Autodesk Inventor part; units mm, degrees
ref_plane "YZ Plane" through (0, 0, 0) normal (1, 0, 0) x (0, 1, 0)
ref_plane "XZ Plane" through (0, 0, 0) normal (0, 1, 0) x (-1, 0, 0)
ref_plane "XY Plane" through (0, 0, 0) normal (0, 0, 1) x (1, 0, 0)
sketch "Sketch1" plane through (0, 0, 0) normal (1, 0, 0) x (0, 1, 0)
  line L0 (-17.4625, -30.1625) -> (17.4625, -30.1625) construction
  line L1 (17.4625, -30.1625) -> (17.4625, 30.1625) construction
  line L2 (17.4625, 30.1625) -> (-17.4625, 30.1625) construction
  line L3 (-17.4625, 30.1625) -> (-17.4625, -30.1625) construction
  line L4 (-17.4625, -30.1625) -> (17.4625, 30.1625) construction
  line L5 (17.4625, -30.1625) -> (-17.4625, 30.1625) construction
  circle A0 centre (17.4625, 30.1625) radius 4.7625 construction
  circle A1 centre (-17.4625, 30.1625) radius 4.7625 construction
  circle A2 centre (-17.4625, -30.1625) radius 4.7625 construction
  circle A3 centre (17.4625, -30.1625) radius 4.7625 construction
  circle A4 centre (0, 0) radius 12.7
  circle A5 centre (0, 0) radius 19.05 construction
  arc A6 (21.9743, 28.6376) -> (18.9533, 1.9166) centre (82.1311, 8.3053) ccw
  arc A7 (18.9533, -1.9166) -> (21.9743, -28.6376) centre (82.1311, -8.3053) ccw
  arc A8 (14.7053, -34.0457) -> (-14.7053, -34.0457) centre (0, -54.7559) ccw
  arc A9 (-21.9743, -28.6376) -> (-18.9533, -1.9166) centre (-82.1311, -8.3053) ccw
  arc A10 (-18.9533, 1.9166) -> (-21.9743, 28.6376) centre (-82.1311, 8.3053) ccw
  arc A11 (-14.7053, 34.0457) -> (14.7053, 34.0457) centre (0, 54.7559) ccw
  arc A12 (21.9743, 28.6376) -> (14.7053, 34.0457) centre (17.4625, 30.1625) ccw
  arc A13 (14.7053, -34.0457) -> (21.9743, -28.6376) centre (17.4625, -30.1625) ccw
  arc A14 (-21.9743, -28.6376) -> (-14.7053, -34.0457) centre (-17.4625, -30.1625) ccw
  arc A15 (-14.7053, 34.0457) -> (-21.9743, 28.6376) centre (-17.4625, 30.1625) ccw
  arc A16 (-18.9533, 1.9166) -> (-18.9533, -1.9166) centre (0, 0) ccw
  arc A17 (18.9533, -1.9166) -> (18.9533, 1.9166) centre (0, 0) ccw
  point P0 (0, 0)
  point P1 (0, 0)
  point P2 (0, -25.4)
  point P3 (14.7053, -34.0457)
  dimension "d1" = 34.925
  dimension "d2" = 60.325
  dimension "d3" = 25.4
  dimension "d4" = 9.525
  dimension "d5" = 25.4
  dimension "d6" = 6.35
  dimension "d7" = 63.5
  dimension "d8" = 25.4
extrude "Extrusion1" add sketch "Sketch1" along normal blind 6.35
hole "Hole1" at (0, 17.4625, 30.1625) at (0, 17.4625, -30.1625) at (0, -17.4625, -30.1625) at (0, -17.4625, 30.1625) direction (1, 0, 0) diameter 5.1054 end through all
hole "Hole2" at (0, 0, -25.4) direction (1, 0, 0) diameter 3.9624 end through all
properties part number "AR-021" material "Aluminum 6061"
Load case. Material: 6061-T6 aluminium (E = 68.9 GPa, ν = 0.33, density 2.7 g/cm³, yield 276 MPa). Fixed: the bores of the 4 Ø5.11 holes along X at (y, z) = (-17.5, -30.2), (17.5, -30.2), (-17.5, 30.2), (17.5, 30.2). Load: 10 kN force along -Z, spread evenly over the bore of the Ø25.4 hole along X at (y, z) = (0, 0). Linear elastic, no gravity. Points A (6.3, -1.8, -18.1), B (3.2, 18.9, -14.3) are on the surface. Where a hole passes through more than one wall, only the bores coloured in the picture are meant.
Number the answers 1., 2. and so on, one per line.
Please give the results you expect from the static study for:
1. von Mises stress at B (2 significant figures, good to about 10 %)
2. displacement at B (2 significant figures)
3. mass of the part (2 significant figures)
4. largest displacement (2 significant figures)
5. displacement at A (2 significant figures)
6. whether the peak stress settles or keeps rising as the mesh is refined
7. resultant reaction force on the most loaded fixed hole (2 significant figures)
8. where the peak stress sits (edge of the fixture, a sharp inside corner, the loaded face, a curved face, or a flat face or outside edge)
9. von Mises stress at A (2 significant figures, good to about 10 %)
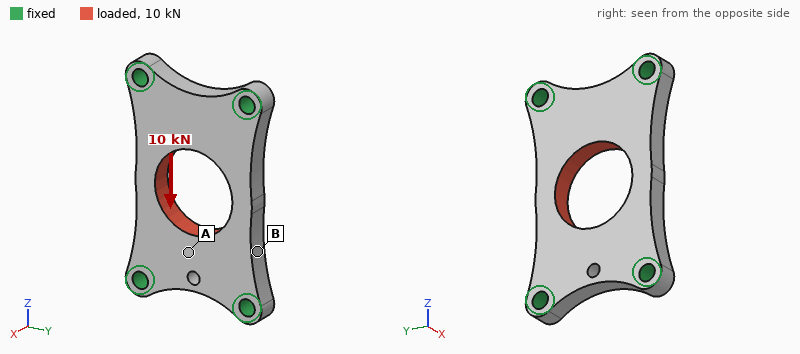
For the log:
1. 29 MPa
2. 6.0 µm
3. 33 g
4. 11 µm
5. 9.8 µm
6. keeps rising
7. 2.7 kN
8. edge of the fixture
9. 15 MPa
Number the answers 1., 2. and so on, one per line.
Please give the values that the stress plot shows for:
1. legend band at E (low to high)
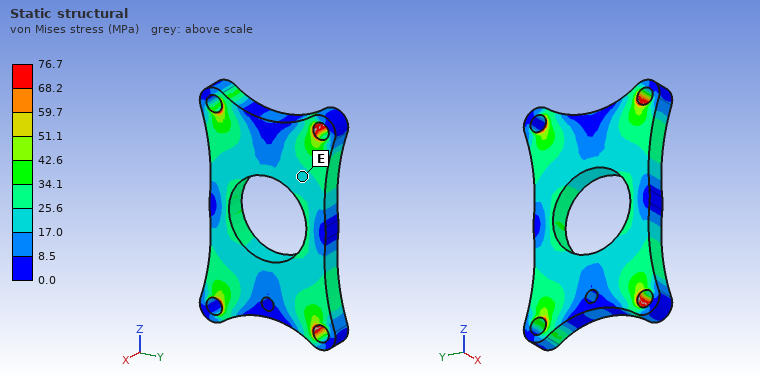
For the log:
1. 17.0 to 25.6 MPa
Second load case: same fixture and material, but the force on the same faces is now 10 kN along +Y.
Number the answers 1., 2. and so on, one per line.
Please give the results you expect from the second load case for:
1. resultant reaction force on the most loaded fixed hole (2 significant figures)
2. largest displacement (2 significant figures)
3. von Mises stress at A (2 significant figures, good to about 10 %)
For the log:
1. 3.2 kN
2. 38 µm
3. 68 MPa
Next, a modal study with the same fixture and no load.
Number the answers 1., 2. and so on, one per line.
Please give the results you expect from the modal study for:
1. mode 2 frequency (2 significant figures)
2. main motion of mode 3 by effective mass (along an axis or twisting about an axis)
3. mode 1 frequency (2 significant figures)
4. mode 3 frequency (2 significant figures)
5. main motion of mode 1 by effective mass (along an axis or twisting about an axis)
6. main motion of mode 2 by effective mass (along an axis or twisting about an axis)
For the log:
1. 12 kHz
2. twisting about Y
3. 8900 Hz
4. 16 kHz
5. along X
6. twisting about Z
